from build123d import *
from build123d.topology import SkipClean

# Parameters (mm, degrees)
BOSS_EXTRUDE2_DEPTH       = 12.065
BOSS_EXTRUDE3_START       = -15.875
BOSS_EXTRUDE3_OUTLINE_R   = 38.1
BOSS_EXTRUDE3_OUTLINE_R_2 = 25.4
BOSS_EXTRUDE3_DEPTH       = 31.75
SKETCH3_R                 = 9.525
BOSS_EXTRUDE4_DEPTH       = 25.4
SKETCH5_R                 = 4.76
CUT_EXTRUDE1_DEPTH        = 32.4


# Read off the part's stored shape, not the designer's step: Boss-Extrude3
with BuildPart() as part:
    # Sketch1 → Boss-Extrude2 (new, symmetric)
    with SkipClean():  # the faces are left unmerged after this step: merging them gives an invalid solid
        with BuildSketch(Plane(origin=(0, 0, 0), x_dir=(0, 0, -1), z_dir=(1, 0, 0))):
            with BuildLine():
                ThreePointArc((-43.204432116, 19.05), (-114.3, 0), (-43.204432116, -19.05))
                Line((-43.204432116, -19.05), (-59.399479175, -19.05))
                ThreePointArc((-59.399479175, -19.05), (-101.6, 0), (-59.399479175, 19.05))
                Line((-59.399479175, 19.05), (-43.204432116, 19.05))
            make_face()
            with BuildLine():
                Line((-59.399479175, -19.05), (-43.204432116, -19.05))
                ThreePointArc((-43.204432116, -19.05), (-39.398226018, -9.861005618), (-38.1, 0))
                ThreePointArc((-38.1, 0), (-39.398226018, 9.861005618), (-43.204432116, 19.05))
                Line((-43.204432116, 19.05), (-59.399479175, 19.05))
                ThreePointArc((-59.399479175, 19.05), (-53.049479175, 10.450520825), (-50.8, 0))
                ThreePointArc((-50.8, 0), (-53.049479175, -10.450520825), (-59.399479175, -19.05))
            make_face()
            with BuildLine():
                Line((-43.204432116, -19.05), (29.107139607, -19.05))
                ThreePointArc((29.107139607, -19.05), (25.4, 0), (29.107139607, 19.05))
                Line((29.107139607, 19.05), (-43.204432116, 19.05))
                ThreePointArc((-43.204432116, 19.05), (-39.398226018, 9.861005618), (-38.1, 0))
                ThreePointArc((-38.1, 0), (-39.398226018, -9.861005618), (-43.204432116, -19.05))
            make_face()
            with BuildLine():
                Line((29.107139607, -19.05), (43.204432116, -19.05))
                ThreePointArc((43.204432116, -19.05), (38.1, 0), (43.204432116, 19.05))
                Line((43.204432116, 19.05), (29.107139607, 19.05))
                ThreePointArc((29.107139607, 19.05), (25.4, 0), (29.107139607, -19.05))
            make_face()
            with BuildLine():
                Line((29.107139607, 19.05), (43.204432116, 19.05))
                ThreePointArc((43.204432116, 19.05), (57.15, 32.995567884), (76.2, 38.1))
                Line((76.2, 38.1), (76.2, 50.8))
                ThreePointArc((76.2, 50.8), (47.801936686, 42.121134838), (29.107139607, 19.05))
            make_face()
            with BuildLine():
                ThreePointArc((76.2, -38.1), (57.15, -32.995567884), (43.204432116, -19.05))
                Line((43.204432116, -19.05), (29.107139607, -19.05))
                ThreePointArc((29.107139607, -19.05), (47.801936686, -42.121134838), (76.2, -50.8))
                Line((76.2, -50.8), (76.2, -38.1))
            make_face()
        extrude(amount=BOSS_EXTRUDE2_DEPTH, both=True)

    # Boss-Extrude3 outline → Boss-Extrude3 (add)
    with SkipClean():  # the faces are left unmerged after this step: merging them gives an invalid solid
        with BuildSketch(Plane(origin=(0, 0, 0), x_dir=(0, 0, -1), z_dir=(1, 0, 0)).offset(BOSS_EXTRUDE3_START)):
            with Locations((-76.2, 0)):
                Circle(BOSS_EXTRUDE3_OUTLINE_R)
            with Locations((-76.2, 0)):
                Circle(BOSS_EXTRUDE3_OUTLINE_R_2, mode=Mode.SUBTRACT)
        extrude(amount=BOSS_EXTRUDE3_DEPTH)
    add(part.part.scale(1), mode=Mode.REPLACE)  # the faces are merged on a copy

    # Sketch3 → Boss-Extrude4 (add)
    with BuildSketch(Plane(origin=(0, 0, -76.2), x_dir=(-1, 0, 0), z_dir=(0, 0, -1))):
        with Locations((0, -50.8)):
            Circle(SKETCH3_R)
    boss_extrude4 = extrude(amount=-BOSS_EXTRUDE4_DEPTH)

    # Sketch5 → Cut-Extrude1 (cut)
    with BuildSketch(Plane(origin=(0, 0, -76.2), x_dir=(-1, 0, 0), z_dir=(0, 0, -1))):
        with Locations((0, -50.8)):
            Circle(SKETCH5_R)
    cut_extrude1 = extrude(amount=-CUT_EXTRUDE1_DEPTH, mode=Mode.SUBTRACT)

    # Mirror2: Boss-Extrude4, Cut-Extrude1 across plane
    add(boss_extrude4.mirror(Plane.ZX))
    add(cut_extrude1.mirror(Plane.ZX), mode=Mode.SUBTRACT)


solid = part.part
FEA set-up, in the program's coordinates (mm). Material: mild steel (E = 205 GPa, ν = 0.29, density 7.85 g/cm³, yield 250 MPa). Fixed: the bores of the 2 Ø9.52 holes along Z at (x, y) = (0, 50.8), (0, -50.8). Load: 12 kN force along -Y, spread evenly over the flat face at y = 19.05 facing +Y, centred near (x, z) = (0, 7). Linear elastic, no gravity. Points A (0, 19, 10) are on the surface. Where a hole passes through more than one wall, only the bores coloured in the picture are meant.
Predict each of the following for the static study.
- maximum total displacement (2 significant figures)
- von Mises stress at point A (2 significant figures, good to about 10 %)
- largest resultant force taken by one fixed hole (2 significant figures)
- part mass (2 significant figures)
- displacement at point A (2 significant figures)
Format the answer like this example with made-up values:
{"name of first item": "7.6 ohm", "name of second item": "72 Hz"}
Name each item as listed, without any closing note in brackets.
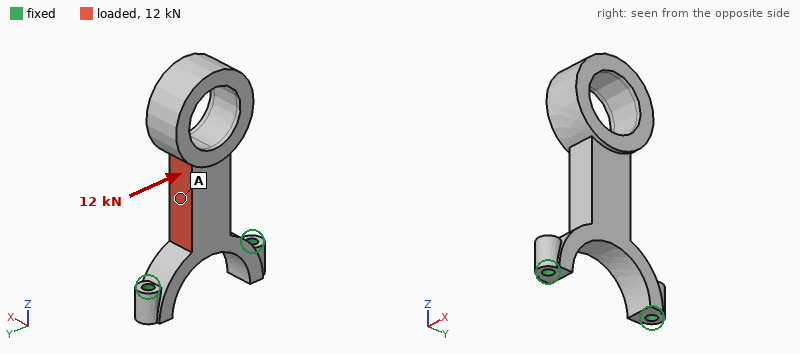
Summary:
{"maximum total displacement": "0.20 mm", "von Mises stress at point A": "18 MPa", "largest resultant force taken by one fixed hole": "12 kN", "part mass": "1.5 kg", "displacement at point A": "0.060 mm"}
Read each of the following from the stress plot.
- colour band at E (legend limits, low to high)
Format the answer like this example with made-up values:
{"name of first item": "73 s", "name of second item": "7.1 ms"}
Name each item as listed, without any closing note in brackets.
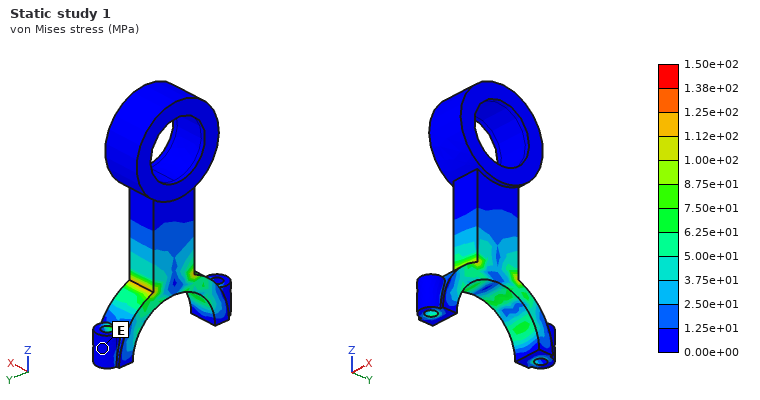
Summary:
{"colour band at E": "0.00e+00 to 1.25e+01 MPa"}
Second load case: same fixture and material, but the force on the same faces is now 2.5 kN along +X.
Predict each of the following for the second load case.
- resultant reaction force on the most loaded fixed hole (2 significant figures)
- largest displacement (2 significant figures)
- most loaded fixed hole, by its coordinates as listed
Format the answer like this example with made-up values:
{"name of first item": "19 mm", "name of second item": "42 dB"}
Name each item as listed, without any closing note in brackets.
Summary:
{"resultant reaction force on the most loaded fixed hole": "1.9 kN", "largest displacement": "0.30 mm", "most loaded fixed hole, by its coordinates as listed": "(0, 50.8)"}
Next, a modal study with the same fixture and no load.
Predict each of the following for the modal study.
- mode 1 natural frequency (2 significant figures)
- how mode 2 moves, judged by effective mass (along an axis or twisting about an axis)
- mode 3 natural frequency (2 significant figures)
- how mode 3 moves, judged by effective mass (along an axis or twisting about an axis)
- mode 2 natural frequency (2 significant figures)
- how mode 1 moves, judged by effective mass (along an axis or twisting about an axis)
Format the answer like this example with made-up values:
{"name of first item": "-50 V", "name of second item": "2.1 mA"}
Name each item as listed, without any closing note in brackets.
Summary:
{"mode 1 natural frequency": "380 Hz", "how mode 2 moves, judged by effective mass": "along Y", "mode 3 natural frequency": "2200 Hz", "how mode 3 moves, judged by effective mass": "twisting about Z", "mode 2 natural frequency": "820 Hz", "how mode 1 moves, judged by effective mass": "along X"}
